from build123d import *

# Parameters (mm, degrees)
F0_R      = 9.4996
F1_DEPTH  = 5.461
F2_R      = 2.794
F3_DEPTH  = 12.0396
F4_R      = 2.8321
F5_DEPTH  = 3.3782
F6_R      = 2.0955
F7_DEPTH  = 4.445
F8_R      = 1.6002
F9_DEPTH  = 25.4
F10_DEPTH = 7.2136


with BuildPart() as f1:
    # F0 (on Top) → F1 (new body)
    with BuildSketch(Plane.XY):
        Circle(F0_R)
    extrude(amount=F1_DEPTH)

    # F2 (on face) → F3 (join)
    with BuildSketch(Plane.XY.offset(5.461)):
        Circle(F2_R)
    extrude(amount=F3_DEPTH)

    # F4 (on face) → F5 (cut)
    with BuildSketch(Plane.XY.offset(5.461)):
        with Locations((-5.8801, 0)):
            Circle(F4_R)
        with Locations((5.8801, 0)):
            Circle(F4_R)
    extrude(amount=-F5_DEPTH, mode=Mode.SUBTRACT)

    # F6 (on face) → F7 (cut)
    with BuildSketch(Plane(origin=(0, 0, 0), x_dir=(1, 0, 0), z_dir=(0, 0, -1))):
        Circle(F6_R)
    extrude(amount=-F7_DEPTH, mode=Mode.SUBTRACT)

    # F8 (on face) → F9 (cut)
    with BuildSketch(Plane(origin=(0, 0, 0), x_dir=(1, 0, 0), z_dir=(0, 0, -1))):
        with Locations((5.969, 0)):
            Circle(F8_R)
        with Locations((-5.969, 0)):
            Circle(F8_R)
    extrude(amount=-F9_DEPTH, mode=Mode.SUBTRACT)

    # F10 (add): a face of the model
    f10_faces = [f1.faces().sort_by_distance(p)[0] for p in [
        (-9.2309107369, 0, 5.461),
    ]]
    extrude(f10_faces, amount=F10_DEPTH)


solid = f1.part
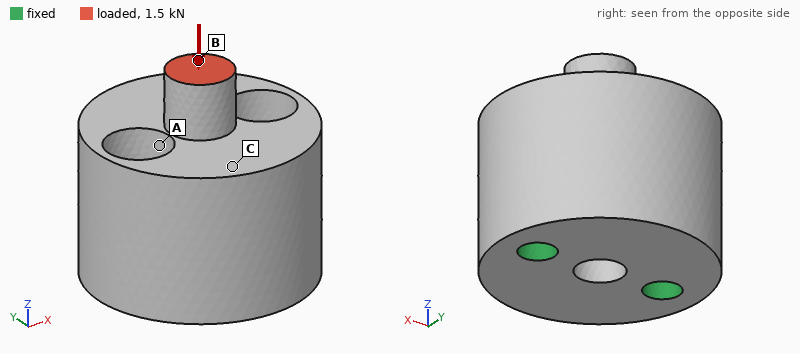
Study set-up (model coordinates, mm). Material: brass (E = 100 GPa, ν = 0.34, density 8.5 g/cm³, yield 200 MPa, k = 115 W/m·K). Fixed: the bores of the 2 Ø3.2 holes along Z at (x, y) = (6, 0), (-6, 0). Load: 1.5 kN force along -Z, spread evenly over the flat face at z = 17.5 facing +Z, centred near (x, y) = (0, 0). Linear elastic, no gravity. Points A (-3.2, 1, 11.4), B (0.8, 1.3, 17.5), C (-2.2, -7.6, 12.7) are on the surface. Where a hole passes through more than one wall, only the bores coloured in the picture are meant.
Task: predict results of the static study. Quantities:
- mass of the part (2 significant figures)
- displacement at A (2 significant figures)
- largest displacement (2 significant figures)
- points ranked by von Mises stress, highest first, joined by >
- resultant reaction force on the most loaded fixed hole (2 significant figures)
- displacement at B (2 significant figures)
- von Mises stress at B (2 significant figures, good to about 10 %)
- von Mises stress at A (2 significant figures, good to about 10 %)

26 g
4.4 µm
8.0 µm
B > A > C
760 N
8.0 µm
62 MPa
36 MPa
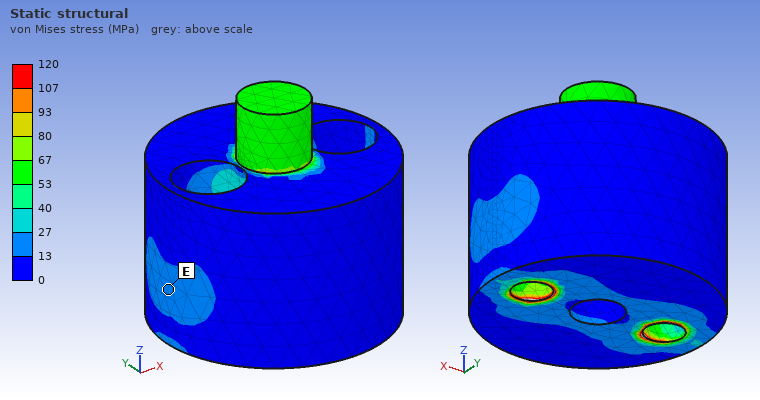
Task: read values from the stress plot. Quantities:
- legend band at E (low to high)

13 to 27 MPa
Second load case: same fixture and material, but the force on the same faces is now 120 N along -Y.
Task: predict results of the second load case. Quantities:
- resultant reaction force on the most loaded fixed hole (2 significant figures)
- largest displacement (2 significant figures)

60 N
15 µm
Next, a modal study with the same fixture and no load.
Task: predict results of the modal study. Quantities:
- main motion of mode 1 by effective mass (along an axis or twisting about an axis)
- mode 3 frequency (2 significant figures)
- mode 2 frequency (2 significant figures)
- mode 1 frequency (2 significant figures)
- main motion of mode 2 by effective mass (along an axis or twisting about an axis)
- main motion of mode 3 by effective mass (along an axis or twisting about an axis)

along Y
23 kHz
16 kHz
6000 Hz
along X
along Z
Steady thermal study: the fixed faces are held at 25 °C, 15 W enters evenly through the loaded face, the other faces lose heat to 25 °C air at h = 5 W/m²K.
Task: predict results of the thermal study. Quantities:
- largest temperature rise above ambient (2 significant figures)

46 K
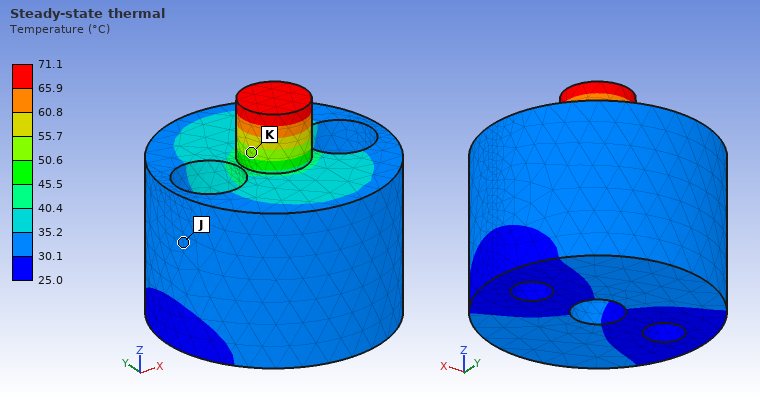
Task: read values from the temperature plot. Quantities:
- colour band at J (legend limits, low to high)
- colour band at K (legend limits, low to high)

30.1 to 35.2 °C
50.6 to 55.7 °C
